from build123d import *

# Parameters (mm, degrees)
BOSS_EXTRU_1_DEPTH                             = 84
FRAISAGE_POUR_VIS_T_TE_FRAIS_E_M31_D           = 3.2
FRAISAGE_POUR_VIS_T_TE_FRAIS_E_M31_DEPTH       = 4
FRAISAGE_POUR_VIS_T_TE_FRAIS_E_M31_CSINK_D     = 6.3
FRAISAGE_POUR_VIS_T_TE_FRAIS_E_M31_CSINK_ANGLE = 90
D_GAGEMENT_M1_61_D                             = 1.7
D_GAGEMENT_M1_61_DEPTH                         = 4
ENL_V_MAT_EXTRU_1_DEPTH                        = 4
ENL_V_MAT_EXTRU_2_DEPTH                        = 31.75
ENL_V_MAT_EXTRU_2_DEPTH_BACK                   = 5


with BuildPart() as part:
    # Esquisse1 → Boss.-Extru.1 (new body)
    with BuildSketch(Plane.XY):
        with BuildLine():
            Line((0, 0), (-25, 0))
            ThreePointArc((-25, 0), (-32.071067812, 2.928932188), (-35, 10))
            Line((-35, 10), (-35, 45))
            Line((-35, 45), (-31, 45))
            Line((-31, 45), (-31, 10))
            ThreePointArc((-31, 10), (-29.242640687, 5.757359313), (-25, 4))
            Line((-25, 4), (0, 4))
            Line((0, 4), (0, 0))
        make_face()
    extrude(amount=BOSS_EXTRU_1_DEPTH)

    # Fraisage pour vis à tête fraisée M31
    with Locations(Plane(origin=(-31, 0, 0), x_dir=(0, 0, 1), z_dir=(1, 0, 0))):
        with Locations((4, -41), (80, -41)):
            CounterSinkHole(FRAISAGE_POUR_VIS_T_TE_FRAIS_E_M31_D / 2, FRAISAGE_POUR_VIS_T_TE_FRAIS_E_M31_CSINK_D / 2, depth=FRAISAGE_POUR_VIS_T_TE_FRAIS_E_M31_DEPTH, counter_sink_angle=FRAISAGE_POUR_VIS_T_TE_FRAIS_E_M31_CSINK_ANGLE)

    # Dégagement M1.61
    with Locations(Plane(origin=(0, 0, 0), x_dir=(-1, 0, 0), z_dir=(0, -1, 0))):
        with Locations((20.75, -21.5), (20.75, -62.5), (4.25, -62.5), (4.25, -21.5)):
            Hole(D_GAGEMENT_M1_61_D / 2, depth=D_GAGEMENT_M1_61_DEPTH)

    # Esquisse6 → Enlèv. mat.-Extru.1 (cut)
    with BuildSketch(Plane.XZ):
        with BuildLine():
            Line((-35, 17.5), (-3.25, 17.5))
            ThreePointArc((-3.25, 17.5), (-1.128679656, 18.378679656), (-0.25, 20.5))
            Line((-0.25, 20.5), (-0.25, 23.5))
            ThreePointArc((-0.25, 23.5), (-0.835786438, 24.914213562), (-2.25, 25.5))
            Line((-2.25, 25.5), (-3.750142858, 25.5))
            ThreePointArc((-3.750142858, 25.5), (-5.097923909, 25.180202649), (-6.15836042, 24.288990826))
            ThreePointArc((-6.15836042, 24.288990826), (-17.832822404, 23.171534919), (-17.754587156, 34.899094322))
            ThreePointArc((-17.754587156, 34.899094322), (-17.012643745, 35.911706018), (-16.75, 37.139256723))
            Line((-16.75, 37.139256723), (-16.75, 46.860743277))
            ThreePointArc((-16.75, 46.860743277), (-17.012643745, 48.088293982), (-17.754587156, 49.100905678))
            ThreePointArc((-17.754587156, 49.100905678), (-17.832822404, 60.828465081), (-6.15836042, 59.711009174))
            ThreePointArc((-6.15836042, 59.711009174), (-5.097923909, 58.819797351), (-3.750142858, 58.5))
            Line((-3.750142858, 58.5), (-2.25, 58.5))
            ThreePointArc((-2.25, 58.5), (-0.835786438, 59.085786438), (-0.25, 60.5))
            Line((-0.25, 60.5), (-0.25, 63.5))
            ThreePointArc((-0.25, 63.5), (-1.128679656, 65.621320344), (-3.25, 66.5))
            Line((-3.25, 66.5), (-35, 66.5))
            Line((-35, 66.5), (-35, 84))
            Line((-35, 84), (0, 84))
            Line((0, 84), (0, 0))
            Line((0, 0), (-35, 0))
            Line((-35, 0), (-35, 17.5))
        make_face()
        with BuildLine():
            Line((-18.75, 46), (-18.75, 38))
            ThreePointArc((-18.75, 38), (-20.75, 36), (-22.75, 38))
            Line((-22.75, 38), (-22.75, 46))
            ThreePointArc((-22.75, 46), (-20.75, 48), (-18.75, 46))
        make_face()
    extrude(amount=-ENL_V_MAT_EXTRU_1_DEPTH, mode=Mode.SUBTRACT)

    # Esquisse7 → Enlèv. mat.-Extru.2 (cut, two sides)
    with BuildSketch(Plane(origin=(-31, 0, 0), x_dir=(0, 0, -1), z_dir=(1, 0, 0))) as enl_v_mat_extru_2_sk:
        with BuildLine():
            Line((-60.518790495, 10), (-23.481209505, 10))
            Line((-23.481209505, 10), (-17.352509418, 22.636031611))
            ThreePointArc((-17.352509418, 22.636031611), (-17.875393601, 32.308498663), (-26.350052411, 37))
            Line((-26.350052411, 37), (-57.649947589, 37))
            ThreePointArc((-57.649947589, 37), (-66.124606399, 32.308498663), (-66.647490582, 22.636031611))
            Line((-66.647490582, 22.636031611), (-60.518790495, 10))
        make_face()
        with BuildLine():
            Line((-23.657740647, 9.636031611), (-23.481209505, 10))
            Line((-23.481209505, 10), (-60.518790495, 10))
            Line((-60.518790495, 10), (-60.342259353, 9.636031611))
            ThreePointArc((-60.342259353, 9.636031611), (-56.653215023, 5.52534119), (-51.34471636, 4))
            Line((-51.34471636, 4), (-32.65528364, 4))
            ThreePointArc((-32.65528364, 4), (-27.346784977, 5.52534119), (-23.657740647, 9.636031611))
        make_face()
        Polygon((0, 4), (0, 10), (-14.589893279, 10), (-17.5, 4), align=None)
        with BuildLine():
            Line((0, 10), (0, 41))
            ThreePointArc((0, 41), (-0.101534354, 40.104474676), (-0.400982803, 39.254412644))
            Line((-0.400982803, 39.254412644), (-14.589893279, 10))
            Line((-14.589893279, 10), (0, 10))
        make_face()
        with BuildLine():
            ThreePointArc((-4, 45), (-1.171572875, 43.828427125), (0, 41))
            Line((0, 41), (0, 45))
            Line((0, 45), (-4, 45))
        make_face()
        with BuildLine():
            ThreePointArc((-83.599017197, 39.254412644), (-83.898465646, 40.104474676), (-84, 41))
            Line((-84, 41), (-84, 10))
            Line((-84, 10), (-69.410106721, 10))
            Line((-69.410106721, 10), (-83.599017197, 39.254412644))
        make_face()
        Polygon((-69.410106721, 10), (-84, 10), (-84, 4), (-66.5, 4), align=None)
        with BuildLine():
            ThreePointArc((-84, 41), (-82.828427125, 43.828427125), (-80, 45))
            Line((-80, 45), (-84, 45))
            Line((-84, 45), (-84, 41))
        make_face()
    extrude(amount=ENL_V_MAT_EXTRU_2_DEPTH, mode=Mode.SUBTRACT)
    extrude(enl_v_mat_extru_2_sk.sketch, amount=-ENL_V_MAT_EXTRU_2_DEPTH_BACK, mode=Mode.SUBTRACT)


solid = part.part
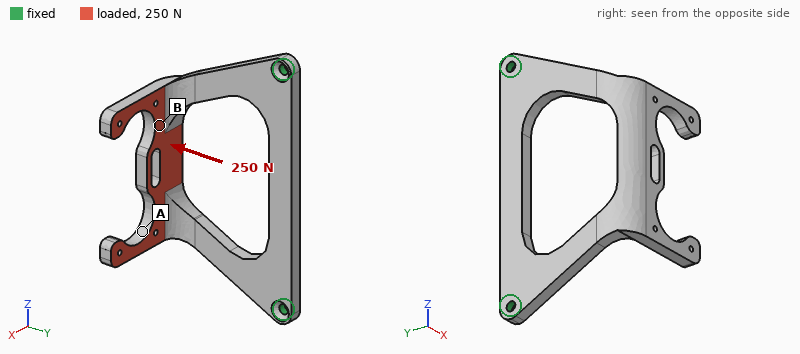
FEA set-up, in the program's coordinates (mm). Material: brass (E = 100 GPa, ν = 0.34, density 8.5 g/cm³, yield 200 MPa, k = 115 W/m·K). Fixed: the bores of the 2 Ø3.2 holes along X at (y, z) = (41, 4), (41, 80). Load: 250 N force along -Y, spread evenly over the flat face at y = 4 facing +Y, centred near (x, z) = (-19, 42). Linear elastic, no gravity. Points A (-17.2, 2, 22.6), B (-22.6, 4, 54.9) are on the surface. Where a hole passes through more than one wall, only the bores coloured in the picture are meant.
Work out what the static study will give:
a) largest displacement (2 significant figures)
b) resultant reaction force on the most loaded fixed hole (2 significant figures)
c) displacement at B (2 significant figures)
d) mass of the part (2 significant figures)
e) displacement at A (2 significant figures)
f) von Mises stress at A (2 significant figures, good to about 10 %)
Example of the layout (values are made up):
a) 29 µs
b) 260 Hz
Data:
a) 0.63 mm
b) 140 N
c) 0.31 mm
d) 72 g
e) 0.38 mm
f) 23 MPa
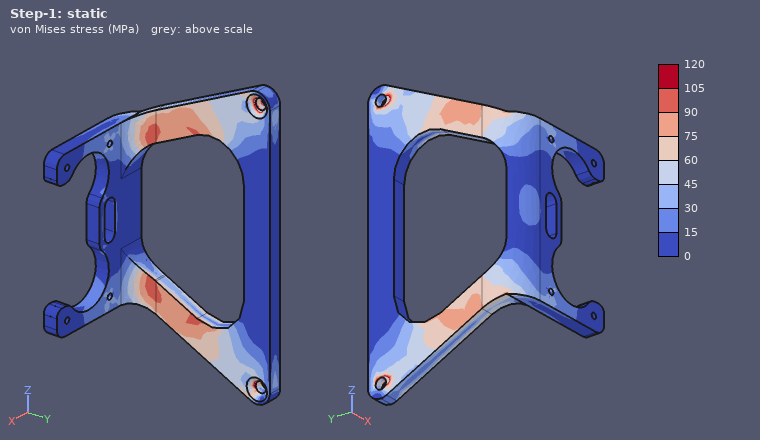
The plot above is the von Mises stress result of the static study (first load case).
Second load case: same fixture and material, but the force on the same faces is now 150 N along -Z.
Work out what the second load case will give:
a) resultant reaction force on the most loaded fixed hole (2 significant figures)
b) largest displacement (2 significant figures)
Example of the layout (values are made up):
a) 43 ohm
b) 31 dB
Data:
a) 99 N
b) 0.11 mm
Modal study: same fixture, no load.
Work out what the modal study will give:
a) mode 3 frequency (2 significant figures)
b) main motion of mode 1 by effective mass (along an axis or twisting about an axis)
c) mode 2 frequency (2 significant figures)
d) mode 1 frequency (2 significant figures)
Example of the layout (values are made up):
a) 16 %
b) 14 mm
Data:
a) 1700 Hz
b) along X
c) 1200 Hz
d) 530 Hz
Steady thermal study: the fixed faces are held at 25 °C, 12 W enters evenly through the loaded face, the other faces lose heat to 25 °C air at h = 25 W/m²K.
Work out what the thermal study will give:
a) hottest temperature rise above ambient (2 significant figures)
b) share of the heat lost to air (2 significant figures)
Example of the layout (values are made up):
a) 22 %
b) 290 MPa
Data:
a) 59 K
b) 31 %
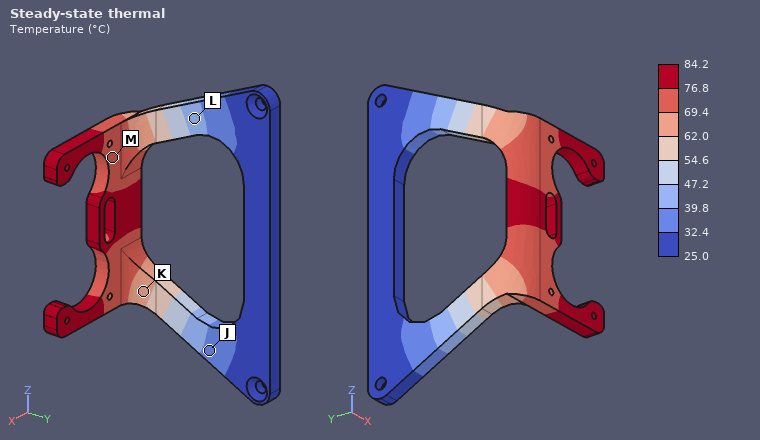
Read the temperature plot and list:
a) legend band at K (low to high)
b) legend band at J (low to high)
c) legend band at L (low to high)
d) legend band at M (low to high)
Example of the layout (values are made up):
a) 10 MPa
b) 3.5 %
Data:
a) 62.0 to 69.4 °C
b) 32.4 to 39.8 °C
c) 39.8 to 47.2 °C
d) 69.4 to 76.8 °C
